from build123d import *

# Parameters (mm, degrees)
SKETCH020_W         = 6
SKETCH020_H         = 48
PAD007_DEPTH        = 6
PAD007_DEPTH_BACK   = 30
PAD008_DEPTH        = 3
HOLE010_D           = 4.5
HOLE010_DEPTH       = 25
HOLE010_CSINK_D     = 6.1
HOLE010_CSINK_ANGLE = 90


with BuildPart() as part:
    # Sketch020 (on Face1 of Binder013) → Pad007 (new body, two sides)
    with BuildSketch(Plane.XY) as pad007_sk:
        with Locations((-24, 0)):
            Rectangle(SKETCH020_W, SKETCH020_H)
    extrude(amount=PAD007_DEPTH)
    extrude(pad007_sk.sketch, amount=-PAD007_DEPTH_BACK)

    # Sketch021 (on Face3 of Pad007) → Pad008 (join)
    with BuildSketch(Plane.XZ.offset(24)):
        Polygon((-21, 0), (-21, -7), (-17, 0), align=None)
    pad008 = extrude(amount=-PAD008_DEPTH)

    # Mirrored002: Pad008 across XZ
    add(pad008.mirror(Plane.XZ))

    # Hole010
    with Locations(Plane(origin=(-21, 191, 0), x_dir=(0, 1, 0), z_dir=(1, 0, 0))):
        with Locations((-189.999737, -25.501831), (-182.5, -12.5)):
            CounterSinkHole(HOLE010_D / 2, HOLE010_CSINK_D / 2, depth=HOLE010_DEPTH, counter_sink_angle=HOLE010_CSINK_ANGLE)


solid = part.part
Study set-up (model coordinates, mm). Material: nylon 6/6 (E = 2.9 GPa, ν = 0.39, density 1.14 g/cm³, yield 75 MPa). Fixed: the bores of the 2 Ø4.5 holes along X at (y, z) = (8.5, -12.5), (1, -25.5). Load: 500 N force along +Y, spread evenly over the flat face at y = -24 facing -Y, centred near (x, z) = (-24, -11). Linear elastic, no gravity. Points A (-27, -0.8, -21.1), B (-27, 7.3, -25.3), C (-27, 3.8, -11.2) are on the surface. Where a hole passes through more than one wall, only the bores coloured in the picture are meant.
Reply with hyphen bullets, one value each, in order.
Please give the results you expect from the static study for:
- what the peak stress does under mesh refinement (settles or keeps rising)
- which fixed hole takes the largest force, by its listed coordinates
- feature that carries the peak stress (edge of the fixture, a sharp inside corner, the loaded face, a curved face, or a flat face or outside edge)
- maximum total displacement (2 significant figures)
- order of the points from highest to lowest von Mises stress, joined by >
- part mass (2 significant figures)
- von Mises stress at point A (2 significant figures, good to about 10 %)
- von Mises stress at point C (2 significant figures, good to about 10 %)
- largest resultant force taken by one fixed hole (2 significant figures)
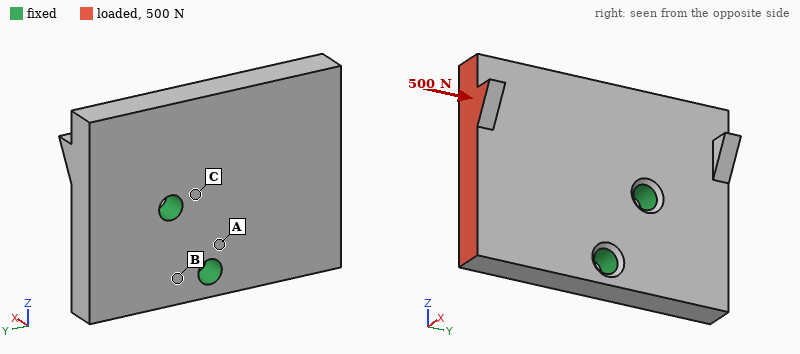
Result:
- keeps rising
- (8.5, -12.5)
- edge of the fixture
- 0.12 mm
- C > A > B
- 12 g
- 2.7 MPa
- 5.5 MPa
- 450 N
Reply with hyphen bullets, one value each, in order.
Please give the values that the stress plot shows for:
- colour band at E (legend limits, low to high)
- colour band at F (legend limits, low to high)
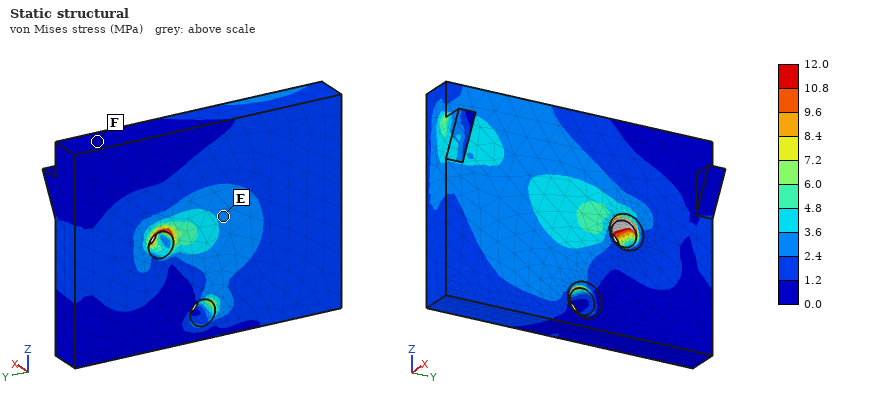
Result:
- 2.4 to 3.6 MPa
- 0.0 to 1.2 MPa
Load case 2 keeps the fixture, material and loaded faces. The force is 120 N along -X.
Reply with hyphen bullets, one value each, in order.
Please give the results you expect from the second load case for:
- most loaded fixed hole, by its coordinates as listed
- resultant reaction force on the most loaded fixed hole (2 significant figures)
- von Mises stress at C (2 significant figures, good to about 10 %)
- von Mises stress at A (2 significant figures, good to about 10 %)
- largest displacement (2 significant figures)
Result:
- (1, -25.5)
- 100 N
- 15 MPa
- 16 MPa
- 0.72 mm
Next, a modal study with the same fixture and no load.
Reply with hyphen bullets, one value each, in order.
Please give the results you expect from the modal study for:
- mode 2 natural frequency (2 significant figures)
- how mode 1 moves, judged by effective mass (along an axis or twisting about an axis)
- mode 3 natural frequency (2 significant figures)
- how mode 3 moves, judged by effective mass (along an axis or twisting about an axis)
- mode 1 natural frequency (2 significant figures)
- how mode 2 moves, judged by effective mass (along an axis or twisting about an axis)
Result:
- 3100 Hz
- along X
- 3900 Hz
- along X
- 1500 Hz
- twisting about Y
